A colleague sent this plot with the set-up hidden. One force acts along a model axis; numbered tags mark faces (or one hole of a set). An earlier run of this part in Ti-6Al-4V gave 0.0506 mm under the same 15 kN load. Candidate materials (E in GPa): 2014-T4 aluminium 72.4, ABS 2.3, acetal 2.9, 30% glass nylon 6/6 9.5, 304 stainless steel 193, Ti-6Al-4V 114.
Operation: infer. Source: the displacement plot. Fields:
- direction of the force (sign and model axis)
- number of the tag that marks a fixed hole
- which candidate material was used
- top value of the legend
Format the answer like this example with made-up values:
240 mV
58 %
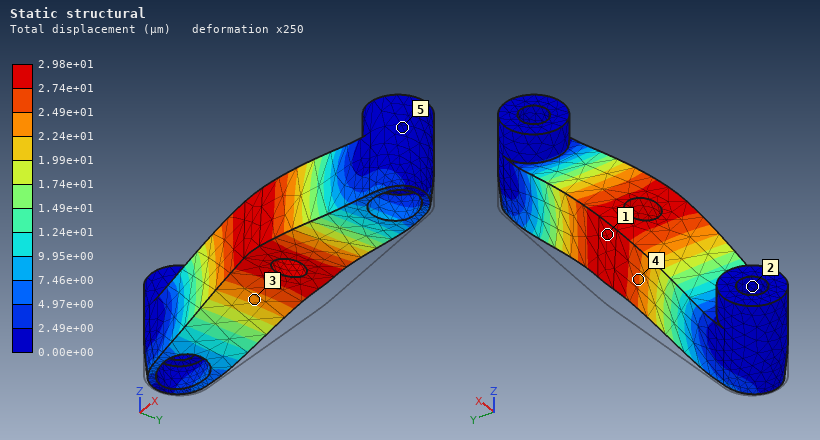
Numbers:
+Z
2
304 stainless steel
2.98e+01 µm
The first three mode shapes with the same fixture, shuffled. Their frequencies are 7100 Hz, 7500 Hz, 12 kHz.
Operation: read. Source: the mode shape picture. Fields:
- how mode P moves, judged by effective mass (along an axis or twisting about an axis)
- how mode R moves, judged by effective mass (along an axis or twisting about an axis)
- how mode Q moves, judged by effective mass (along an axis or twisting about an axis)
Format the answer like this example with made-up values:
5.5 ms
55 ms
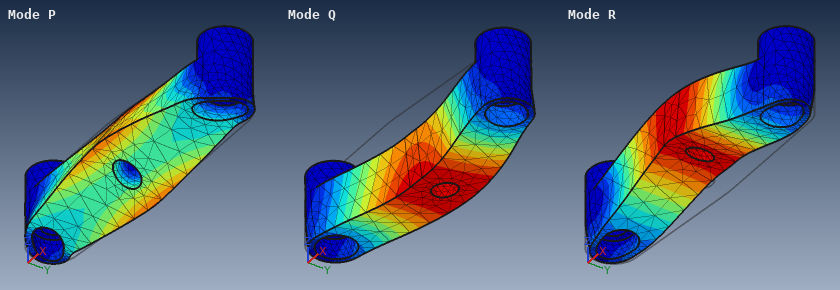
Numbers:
twisting about X
along Z
along Y
